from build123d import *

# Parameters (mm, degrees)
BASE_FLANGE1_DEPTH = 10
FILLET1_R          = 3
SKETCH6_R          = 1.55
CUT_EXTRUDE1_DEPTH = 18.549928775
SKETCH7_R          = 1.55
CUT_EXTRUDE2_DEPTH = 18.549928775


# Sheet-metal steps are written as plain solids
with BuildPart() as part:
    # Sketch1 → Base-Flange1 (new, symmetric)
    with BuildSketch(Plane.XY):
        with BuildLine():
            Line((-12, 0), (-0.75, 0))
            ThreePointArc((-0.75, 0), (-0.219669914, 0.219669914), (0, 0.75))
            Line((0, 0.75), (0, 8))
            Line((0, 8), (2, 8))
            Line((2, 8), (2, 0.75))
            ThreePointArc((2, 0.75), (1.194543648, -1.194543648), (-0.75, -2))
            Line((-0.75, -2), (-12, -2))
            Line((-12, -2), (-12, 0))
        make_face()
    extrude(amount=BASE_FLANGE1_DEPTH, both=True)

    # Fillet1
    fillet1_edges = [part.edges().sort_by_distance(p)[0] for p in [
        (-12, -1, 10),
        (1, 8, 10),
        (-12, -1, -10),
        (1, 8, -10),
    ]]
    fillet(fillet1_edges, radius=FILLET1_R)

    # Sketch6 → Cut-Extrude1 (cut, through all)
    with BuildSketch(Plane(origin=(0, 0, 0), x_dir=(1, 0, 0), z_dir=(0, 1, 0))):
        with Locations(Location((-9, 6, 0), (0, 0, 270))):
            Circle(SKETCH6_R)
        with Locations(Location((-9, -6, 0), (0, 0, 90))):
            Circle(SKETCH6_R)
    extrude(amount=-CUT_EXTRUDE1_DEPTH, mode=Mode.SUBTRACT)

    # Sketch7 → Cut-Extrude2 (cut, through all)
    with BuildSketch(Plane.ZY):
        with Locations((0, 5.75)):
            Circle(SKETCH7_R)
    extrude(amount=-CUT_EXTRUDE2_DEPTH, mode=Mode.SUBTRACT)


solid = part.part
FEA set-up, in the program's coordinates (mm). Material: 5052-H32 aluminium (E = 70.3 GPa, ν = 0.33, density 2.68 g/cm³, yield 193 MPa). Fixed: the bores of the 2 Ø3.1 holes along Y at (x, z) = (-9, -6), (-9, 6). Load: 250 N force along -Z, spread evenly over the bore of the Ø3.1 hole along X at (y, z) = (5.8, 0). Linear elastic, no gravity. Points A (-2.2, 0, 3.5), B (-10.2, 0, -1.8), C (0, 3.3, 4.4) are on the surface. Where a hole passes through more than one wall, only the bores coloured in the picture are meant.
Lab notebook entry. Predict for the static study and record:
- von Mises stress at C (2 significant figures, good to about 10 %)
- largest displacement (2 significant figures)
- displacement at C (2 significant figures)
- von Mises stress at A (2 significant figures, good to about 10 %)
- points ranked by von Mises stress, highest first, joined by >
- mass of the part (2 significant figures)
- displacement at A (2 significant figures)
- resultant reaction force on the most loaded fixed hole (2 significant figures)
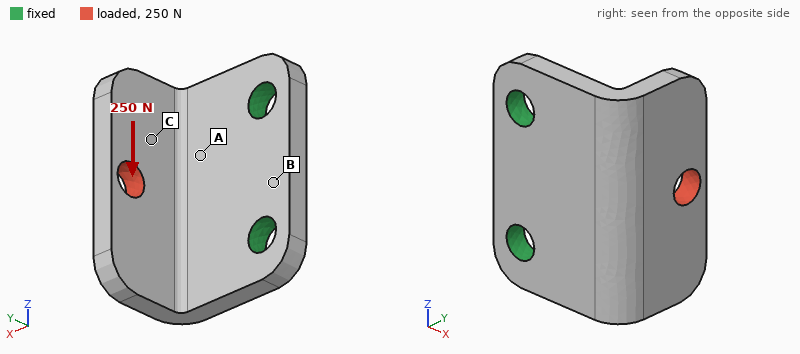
37 MPa
61 µm
31 µm
68 MPa
A > C > B
2.1 g
10 µm
240 N
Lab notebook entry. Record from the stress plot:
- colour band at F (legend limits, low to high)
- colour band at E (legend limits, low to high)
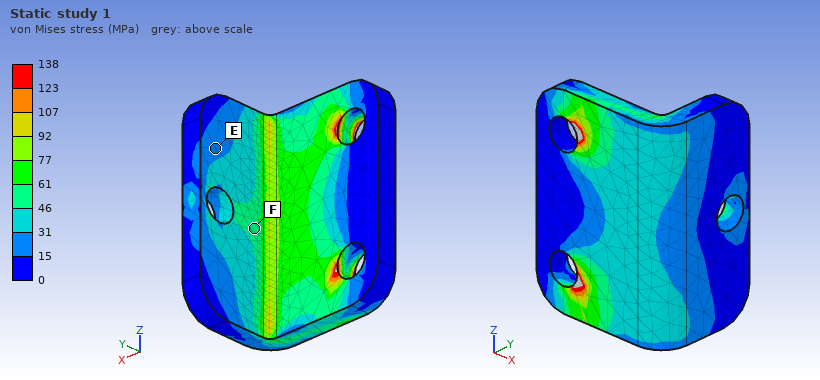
46 to 61 MPa
15 to 31 MPa
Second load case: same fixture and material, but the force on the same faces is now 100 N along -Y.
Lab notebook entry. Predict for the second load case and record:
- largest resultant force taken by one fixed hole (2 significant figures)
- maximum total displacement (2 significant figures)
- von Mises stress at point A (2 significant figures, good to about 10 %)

50 N
53 µm
21 MPa
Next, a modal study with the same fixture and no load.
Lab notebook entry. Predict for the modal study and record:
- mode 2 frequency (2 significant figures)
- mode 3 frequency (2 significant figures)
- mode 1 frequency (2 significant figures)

12 kHz
20 kHz
7200 Hz
